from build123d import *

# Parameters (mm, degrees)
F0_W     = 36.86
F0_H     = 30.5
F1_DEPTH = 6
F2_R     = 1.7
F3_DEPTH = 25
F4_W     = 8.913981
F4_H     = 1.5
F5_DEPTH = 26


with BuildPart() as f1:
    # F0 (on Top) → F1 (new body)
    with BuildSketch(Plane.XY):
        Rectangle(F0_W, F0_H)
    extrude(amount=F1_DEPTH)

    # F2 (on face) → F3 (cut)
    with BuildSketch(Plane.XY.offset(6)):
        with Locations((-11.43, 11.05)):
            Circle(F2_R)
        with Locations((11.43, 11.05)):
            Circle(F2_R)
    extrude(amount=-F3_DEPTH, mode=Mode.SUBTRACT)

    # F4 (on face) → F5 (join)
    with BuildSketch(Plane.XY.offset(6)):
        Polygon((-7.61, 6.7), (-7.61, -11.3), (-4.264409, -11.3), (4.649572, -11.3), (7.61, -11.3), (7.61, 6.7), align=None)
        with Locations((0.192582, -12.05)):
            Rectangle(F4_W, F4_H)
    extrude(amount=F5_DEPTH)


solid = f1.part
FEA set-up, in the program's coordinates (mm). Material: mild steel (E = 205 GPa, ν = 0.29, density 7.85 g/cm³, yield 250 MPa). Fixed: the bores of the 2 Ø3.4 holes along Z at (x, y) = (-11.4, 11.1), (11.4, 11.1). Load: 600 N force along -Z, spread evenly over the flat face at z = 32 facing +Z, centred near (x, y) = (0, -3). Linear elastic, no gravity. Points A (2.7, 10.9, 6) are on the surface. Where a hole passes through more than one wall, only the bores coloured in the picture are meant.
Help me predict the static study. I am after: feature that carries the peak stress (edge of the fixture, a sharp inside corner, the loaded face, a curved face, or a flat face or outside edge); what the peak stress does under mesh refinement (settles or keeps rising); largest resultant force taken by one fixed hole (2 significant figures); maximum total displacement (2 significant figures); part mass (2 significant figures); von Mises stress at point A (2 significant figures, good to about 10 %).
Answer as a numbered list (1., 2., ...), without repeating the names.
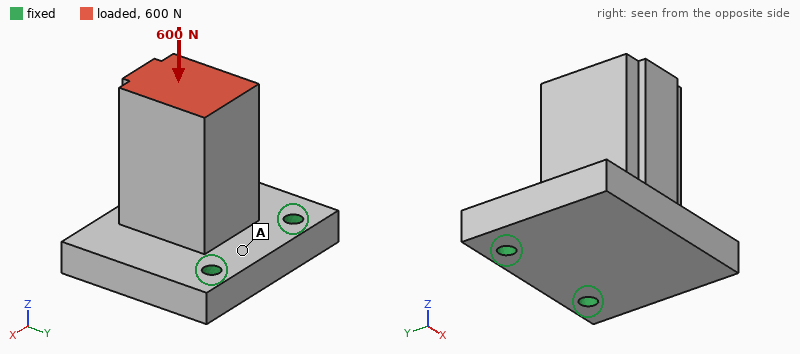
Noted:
1. edge of the fixture
2. keeps rising
3. 300 N
4. 18 µm
5. 110 g
6. 10 MPa
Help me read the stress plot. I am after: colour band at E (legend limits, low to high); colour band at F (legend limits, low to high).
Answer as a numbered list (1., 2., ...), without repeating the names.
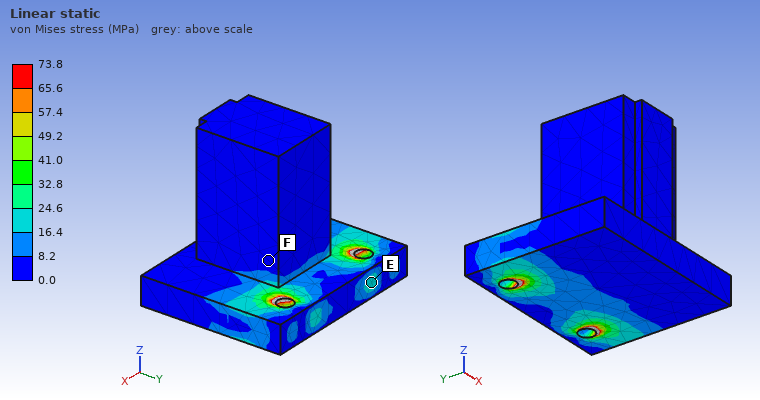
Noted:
1. 16.4 to 24.6 MPa
2. 0.0 to 8.2 MPa
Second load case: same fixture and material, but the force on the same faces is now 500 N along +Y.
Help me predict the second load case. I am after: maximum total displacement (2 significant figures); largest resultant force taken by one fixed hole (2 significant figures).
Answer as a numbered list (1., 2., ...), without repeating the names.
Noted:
1. 43 µm
2. 280 N
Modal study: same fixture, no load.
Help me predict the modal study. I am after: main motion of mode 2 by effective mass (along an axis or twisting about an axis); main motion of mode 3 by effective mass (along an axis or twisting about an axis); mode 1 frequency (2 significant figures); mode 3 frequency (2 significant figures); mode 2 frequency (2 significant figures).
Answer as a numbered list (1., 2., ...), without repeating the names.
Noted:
1. along X
2. along Z
3. 3100 Hz
4. 14 kHz
5. 6700 Hz
